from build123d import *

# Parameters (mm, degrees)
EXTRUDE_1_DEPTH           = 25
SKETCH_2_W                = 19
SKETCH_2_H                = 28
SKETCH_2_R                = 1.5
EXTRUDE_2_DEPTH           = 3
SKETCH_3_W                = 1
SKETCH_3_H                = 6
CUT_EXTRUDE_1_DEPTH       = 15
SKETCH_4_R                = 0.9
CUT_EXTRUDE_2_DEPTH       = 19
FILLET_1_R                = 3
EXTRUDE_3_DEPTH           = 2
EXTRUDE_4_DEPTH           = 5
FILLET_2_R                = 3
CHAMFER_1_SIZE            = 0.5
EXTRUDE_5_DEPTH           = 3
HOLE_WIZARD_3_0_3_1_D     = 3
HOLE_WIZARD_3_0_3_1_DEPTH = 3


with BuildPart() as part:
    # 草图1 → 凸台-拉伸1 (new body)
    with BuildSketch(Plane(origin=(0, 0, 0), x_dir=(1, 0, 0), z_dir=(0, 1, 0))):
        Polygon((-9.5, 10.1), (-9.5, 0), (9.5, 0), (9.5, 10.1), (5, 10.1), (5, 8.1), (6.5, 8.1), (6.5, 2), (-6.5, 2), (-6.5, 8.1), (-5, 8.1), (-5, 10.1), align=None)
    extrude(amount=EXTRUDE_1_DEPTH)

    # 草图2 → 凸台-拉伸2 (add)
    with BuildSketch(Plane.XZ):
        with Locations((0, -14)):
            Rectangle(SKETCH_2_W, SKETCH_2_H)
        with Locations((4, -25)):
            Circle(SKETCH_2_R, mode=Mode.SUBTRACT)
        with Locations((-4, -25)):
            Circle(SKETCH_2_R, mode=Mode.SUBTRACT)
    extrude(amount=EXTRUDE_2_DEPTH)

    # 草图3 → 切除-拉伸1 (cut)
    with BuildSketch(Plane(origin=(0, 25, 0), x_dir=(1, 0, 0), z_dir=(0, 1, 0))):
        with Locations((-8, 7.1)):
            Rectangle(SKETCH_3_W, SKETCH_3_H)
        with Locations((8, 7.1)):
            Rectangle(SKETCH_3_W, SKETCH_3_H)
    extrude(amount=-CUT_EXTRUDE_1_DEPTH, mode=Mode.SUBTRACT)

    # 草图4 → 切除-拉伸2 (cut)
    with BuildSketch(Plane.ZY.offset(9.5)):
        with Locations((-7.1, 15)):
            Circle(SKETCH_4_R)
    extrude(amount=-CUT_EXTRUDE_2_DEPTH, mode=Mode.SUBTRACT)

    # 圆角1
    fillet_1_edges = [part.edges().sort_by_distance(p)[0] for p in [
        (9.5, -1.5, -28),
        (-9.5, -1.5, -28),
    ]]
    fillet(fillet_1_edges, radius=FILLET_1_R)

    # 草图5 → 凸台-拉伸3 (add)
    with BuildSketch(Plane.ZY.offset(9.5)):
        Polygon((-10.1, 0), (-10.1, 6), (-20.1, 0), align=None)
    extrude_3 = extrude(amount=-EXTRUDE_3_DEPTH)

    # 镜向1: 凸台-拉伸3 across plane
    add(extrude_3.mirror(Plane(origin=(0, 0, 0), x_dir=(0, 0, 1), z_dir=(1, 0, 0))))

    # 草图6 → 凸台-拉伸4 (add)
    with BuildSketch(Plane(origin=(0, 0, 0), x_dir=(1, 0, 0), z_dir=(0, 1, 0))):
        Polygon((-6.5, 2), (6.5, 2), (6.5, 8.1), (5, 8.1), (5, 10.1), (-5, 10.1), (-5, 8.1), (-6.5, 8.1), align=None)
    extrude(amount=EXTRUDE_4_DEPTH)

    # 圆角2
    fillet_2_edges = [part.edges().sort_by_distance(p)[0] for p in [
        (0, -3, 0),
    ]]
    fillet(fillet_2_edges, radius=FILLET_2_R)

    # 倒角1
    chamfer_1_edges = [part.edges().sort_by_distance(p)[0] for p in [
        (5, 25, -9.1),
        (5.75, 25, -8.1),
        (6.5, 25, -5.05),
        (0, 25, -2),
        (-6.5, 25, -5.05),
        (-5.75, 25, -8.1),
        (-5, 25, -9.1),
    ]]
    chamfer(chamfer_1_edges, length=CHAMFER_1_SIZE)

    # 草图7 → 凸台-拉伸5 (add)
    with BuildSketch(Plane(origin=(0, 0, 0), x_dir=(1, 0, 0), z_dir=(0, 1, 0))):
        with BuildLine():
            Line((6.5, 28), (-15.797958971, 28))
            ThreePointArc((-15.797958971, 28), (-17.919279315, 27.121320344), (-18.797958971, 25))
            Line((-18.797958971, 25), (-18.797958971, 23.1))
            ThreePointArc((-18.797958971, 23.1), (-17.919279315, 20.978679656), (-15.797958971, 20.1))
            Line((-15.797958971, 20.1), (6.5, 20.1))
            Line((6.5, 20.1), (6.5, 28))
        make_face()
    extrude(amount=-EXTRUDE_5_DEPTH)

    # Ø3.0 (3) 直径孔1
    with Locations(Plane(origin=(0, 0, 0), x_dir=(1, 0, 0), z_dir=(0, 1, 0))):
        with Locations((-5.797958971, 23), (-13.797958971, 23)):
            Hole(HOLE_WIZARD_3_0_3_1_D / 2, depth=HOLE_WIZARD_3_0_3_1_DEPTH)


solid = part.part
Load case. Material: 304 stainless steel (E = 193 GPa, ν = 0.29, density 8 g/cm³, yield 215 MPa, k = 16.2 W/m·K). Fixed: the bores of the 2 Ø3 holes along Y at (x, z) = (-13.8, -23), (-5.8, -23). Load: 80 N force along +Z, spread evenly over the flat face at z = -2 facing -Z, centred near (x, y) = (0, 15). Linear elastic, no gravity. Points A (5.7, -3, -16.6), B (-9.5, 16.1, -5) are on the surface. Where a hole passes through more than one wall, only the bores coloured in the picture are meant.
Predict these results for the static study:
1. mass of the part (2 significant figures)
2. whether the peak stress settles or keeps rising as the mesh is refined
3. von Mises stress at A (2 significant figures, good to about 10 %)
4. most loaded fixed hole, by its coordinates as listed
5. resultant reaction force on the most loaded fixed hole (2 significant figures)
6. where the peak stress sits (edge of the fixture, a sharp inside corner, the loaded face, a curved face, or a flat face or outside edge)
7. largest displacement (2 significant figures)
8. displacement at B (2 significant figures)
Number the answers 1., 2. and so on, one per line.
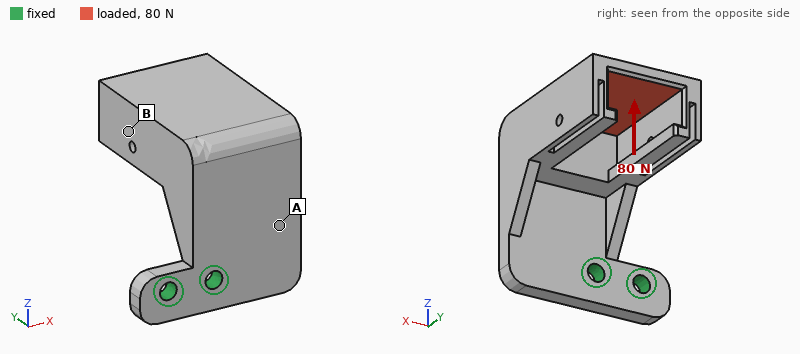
1. 36 g
2. keeps rising
3. 23 MPa
4. (-5.8, -23)
5. 100 N
6. edge of the fixture
7. 55 µm
8. 36 µm
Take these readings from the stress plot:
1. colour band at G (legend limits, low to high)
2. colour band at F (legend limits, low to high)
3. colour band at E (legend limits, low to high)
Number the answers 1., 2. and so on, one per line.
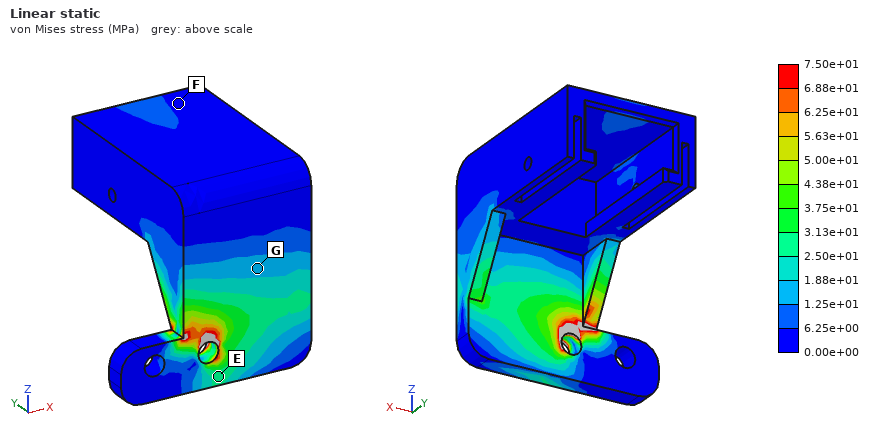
1. 1.25e+01 to 1.88e+01 MPa
2. 0.00e+00 to 6.25e+00 MPa
3. 2.50e+01 to 3.13e+01 MPa
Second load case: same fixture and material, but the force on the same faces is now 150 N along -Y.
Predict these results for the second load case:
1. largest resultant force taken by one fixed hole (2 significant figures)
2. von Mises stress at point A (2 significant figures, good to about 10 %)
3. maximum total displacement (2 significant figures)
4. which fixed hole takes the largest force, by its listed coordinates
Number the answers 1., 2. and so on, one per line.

1. 200 N
2. 35 MPa
3. 0.11 mm
4. (-5.8, -23)
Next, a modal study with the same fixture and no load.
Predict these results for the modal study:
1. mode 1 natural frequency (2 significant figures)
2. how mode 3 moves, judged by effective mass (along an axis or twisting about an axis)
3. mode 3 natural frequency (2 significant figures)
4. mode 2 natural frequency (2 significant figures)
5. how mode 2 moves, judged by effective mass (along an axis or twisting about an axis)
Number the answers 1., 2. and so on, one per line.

1. 1400 Hz
2. along X
3. 5300 Hz
4. 2100 Hz
5. along X
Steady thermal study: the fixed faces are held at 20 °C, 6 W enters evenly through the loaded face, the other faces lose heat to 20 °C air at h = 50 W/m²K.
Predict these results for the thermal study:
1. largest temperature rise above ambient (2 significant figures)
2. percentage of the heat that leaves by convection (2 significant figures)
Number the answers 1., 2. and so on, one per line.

1. 60 K
2. 81 %
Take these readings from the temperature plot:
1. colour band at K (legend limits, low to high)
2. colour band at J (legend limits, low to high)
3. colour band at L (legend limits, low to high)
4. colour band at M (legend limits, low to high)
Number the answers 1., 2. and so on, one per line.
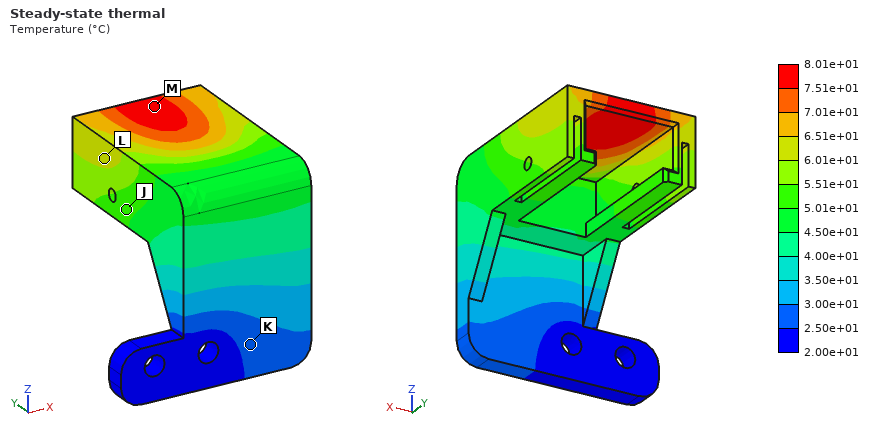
1. 2.50e+01 to 3.00e+01 °C
2. 5.01e+01 to 5.51e+01 °C
3. 6.01e+01 to 6.51e+01 °C
4. 7.51e+01 to 8.01e+01 °C
